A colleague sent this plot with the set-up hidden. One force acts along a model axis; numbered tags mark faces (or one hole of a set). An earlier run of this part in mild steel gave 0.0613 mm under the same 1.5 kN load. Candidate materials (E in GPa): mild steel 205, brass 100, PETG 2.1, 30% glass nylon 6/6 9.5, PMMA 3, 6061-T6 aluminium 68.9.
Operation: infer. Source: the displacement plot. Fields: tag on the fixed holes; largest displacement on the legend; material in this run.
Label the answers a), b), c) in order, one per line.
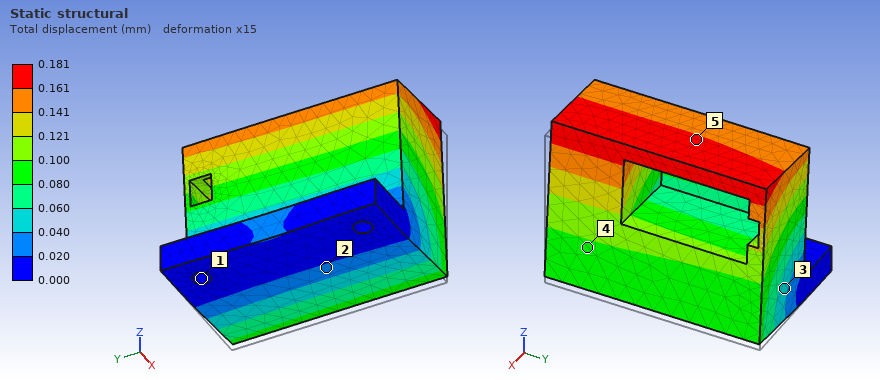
a) 1
b) 0.181 mm
c) 6061-T6 aluminium
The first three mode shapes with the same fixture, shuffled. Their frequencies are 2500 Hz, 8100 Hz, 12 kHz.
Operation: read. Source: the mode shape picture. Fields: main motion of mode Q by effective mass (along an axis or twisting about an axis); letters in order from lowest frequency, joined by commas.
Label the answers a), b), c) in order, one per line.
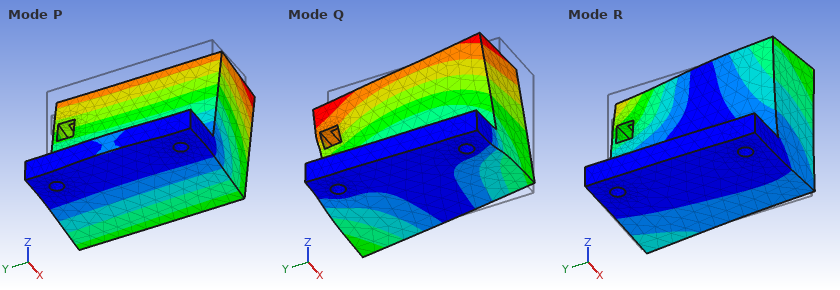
a) along Y
b) P, Q, R
